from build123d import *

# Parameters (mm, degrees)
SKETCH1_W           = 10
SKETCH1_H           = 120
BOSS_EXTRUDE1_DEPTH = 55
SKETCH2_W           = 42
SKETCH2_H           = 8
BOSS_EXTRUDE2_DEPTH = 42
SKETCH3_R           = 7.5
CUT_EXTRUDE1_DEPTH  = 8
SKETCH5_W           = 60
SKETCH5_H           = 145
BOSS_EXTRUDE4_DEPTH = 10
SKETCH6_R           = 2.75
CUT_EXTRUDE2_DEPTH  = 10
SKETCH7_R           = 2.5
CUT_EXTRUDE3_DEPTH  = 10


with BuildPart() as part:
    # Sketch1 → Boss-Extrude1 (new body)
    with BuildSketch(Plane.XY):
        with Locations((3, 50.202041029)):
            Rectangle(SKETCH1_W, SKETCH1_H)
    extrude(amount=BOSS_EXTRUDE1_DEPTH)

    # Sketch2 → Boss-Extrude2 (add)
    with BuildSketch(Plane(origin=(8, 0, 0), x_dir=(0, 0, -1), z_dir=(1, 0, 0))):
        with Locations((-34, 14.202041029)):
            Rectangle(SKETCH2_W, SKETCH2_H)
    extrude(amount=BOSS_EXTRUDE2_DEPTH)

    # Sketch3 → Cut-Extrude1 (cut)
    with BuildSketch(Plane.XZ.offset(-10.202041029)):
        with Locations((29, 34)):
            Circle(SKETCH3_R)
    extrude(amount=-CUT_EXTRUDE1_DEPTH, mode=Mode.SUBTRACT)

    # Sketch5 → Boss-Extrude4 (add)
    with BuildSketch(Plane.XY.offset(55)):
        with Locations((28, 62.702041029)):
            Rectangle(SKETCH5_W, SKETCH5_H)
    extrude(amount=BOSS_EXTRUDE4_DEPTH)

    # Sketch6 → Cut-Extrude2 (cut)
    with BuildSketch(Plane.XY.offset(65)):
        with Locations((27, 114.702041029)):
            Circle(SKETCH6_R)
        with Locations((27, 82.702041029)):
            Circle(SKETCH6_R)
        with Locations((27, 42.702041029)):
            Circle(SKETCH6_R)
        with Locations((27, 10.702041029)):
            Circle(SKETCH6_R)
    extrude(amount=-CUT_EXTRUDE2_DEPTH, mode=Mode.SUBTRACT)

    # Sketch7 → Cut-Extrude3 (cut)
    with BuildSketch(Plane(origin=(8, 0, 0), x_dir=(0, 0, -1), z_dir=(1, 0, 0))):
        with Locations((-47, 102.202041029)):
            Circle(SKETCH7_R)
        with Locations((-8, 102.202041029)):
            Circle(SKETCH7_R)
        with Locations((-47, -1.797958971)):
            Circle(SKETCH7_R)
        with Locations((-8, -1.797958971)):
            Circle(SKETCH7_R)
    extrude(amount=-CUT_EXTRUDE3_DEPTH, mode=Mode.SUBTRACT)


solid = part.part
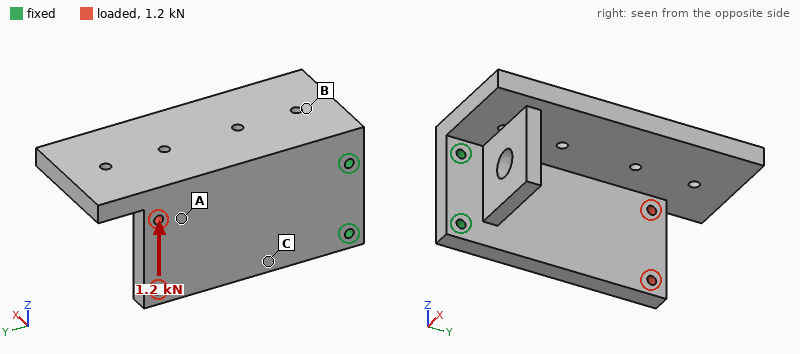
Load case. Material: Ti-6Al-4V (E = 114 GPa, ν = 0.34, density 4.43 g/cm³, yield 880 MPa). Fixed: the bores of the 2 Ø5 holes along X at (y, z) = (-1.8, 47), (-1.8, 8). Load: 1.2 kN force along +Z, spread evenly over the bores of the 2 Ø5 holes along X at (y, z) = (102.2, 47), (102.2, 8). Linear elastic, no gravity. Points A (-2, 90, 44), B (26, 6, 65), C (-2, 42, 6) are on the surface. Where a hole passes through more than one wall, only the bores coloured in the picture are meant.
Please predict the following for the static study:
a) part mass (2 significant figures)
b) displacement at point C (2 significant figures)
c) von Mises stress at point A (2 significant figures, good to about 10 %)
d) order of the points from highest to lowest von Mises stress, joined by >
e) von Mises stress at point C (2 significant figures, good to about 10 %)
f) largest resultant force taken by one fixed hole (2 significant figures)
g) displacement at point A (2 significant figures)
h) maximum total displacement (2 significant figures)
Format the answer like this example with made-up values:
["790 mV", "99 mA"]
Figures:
["730 g", "10 µm", "4.3 MPa", "C > A > B", "7.6 MPa", "3.1 kN", "24 µm", "39 µm"]
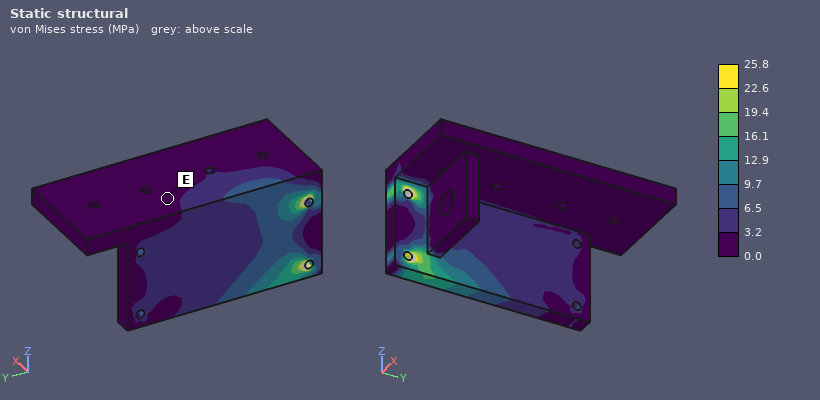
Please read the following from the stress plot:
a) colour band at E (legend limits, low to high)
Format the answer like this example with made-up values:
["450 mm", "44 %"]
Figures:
["0.0 to 3.2 MPa"]
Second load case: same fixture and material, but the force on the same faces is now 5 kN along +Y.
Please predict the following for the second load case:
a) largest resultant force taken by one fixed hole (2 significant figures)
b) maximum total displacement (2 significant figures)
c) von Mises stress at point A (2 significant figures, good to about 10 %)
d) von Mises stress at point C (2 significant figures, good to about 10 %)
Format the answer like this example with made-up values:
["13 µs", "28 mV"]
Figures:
["2.5 kN", "14 µm", "10 MPa", "11 MPa"]
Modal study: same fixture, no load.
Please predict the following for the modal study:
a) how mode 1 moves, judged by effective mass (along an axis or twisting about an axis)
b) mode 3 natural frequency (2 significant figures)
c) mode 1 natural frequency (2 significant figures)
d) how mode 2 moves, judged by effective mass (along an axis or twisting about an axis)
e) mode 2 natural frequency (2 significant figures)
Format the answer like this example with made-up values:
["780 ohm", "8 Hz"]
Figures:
["along X", "2200 Hz", "490 Hz", "along Z", "1200 Hz"]
